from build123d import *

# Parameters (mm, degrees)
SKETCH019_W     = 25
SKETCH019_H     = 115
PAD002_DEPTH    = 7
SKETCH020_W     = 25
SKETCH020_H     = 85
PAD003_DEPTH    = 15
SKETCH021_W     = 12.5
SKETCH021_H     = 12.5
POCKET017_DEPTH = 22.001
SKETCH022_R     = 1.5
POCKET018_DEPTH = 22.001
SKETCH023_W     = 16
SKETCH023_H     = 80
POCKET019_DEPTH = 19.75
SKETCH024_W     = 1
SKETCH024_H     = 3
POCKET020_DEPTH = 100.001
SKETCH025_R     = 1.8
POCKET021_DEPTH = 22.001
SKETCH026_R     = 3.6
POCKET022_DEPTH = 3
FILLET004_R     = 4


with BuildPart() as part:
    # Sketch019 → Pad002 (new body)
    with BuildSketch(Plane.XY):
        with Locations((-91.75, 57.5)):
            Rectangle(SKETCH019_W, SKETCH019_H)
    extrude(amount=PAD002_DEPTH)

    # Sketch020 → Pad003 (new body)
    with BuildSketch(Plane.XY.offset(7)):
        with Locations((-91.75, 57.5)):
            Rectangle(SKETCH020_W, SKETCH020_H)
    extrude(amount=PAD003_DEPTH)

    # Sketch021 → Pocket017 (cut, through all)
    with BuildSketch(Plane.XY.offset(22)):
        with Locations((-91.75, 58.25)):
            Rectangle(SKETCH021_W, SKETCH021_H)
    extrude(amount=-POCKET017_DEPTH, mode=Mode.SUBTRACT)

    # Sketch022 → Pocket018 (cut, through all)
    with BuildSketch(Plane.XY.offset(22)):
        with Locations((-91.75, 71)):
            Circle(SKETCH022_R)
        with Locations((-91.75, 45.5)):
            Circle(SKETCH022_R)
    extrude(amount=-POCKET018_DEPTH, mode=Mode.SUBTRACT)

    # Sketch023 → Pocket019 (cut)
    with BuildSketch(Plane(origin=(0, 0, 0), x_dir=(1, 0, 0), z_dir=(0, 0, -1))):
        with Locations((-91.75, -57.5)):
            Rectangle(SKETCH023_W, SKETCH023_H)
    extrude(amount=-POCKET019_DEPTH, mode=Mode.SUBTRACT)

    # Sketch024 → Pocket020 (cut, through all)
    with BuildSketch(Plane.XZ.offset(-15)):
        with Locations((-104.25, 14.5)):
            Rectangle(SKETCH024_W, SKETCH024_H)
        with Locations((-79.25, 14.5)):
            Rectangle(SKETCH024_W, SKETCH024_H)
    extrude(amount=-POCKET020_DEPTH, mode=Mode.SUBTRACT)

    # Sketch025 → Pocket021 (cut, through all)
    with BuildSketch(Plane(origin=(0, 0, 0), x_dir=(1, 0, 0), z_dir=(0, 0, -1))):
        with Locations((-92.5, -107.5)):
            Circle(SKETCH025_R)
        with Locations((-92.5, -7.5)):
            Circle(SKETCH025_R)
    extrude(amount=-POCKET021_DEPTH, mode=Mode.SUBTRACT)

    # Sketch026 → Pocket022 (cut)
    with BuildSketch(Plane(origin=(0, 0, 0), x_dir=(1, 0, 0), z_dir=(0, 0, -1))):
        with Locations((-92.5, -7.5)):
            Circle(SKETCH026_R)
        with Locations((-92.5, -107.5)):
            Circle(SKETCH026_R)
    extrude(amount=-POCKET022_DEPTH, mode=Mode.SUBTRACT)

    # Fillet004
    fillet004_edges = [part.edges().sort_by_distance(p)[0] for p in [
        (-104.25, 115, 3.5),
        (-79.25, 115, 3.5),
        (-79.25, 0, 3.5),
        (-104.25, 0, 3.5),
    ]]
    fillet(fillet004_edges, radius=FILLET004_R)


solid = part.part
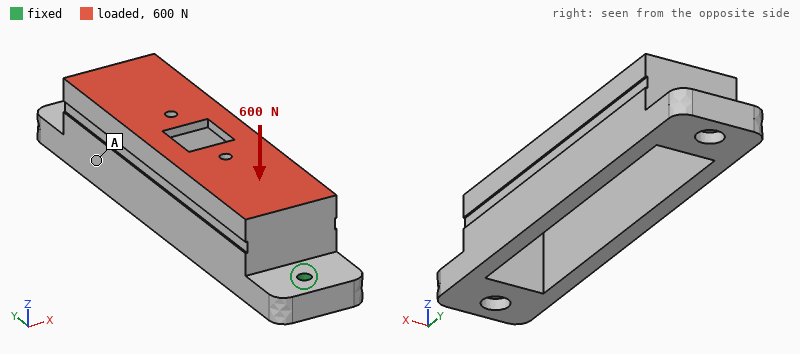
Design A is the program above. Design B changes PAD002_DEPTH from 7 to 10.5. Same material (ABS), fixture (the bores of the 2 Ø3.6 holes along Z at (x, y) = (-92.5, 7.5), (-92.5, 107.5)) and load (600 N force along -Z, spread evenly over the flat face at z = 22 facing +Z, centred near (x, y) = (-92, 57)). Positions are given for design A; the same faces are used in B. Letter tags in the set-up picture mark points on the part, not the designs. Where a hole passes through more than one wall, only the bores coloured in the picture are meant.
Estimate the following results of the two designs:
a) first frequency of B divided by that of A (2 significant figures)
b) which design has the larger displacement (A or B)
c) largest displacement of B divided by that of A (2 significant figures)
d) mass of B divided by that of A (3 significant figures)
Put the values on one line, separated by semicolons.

1.4; A; 0.77; 1.10
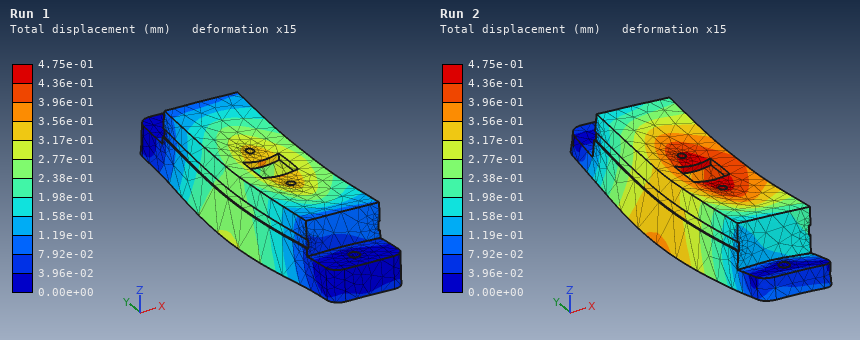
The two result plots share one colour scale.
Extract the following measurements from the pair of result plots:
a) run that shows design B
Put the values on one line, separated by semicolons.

Run 1
